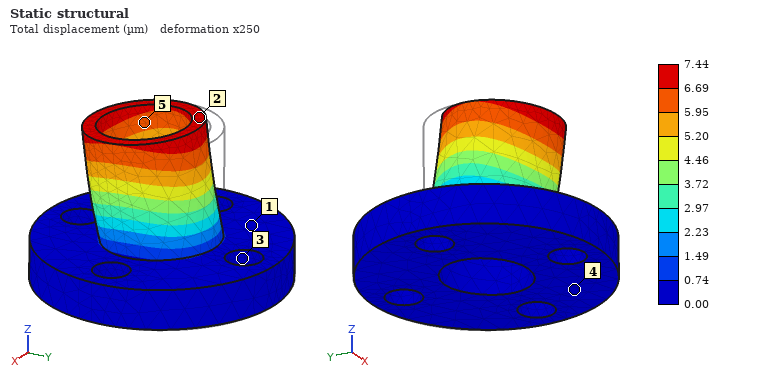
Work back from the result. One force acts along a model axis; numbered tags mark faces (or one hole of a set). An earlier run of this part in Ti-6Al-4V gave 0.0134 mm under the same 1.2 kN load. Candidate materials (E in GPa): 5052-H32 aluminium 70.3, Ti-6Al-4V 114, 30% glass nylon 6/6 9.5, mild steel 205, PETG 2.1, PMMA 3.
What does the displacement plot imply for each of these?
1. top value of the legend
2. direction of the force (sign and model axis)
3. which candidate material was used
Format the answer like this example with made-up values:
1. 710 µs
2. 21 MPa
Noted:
1. 7.44 µm
2. -Y
3. mild steel
